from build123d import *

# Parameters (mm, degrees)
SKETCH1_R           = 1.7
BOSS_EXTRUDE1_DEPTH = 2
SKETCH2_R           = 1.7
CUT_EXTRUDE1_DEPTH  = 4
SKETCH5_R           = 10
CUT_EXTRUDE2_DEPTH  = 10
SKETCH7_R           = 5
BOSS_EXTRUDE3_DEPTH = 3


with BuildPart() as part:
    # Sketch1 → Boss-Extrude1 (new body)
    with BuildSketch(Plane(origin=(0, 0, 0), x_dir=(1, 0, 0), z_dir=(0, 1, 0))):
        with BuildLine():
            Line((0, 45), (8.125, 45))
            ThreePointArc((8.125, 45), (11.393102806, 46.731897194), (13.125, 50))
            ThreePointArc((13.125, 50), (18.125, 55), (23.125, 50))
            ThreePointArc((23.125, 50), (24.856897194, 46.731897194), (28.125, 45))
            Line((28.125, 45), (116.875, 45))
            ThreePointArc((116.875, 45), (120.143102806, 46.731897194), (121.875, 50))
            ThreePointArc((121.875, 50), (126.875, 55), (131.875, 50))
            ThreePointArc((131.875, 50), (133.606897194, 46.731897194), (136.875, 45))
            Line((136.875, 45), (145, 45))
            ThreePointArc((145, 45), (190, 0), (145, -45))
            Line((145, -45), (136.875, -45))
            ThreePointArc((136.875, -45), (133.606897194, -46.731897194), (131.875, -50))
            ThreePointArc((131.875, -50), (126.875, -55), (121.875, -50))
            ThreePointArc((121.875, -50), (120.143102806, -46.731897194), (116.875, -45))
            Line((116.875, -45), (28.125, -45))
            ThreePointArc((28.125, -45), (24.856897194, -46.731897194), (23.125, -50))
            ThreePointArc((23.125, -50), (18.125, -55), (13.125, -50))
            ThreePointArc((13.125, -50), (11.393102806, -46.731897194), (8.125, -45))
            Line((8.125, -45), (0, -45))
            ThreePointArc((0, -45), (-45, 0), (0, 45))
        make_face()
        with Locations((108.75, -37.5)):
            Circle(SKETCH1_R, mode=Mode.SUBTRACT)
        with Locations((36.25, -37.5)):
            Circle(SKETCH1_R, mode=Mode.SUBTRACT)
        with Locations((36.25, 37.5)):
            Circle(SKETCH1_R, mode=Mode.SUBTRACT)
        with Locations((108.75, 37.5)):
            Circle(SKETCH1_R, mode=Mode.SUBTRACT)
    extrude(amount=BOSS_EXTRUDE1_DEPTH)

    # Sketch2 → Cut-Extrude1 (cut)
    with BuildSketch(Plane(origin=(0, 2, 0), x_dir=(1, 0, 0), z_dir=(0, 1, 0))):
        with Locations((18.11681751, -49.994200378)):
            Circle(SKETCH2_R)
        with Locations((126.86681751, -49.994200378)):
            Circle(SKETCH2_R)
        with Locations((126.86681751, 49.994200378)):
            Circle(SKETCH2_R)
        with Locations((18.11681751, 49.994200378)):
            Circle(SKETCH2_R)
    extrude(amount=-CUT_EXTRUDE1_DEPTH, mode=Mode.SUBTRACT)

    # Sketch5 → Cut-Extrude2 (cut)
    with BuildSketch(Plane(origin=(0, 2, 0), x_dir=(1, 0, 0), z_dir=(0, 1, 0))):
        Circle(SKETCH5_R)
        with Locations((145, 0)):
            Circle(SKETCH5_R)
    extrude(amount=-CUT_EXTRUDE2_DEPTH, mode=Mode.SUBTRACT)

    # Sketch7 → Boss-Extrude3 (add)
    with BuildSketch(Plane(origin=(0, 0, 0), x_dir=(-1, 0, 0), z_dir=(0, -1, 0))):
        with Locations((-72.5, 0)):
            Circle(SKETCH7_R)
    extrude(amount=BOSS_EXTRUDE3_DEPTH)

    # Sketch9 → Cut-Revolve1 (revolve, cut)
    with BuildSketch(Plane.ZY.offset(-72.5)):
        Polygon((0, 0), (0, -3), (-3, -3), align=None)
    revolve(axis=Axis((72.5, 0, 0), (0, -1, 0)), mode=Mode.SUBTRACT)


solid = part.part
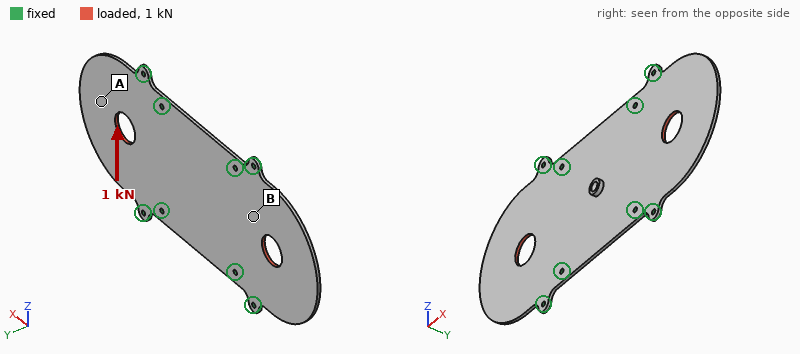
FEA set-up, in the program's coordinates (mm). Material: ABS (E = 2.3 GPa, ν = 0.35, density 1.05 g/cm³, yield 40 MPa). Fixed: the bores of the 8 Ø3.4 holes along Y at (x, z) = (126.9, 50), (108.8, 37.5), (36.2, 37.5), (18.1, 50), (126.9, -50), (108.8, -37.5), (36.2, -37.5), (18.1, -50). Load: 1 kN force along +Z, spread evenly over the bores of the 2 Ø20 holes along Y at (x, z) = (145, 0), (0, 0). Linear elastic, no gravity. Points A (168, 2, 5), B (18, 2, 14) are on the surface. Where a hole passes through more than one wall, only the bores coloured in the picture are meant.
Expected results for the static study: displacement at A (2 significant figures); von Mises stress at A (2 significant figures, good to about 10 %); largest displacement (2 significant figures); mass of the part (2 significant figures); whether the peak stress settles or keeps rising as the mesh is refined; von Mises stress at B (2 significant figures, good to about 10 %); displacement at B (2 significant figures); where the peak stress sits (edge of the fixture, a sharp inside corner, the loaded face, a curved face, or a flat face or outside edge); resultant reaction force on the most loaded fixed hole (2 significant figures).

0.14 mm
1.5 MPa
0.16 mm
40 g
keeps rising
3.5 MPa
0.050 mm
edge of the fixture
170 N
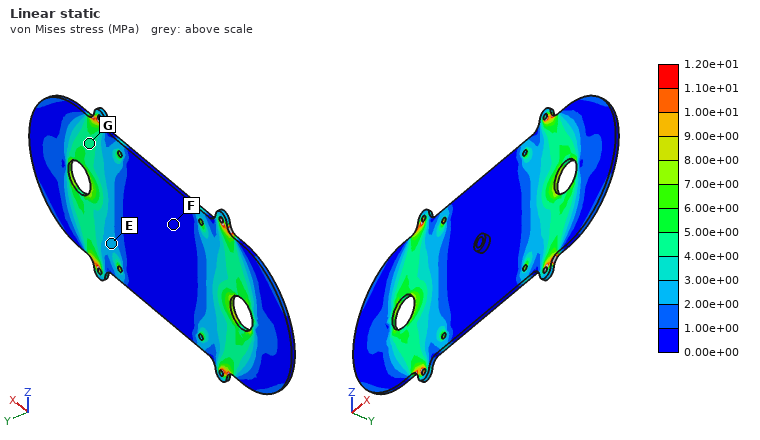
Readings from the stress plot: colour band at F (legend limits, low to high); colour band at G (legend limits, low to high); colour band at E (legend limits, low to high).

0.00e+00 to 1.00e+00 MPa
4.00e+00 to 5.00e+00 MPa
2.00e+00 to 3.00e+00 MPa
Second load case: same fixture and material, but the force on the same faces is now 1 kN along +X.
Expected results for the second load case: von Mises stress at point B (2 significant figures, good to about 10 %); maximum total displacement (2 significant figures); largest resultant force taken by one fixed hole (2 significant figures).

2.9 MPa
0.12 mm
200 N
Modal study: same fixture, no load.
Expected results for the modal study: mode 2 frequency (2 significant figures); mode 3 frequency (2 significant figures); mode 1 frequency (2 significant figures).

100 Hz
310 Hz
100 Hz
